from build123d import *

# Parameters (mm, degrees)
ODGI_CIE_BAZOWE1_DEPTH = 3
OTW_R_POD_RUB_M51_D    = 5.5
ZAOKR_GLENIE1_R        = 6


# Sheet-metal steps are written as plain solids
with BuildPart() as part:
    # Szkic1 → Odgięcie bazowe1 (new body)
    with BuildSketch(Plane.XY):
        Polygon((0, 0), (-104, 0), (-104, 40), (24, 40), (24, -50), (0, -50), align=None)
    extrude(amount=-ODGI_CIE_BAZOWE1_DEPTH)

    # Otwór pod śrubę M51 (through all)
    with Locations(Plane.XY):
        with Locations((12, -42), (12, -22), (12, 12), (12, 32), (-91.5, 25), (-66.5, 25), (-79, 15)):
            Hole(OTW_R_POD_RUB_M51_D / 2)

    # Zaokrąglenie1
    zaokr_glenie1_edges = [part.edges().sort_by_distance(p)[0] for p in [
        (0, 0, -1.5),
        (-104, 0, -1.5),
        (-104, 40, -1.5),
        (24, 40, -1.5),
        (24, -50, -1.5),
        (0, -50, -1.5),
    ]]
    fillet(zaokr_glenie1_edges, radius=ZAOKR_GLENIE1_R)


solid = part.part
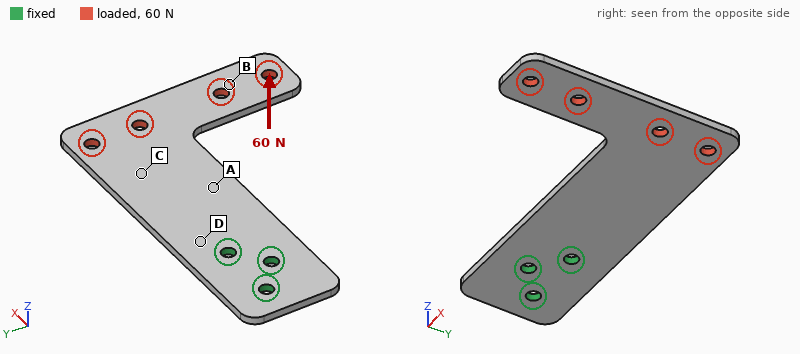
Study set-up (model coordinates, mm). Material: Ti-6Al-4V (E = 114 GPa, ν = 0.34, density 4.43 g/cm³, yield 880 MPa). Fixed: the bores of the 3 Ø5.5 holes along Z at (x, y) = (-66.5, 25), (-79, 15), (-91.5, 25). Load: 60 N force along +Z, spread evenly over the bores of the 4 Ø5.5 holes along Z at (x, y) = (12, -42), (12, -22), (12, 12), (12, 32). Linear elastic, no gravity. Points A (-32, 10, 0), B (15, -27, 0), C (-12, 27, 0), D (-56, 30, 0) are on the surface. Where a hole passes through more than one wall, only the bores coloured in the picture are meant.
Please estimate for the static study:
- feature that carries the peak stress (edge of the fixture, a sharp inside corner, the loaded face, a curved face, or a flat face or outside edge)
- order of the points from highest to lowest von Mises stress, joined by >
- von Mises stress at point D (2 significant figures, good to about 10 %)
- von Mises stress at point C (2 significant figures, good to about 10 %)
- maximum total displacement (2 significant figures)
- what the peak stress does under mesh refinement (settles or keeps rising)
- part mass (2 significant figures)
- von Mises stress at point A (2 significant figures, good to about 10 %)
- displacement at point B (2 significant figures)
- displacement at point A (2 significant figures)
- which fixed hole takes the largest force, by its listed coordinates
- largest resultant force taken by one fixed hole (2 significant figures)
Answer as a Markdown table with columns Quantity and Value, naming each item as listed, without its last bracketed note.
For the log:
| Quantity | Value |
|---|---|
| feature that carries the peak stress | edge of the fixture |
| order of the points from highest to lowest von Mises stress, joined by > | D > A > C > B |
| von Mises stress at point D | 74 MPa |
| von Mises stress at point C | 28 MPa |
| maximum total displacement | 1.9 mm |
| what the peak stress does under mesh refinement | keeps rising |
| part mass | 81 g |
| von Mises stress at point A | 48 MPa |
| displacement at point B | 1.5 mm |
| displacement at point A | 0.28 mm |
| which fixed hole takes the largest force, by its listed coordinates | (-66.5, 25) |
| largest resultant force taken by one fixed hole | 150 N |
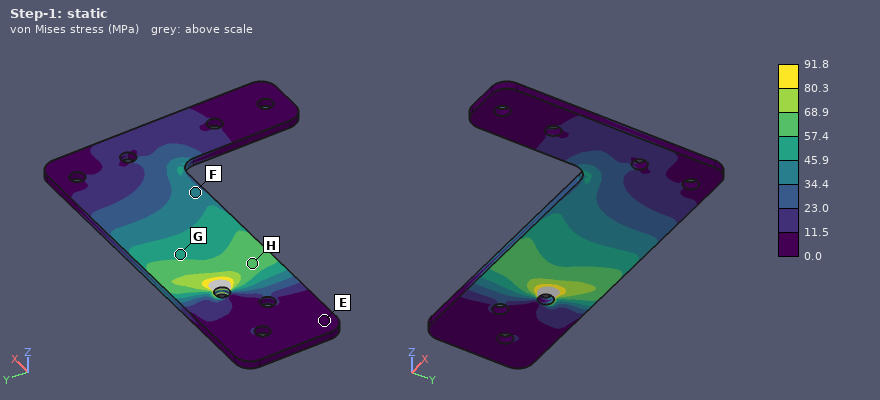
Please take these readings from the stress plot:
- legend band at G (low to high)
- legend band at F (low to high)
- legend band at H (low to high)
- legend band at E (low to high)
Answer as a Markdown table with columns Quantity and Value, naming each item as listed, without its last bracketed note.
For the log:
| Quantity | Value |
|---|---|
| legend band at G | 45.9 to 57.4 MPa |
| legend band at F | 34.4 to 45.9 MPa |
| legend band at H | 57.4 to 68.9 MPa |
| legend band at E | 0.0 to 11.5 MPa |
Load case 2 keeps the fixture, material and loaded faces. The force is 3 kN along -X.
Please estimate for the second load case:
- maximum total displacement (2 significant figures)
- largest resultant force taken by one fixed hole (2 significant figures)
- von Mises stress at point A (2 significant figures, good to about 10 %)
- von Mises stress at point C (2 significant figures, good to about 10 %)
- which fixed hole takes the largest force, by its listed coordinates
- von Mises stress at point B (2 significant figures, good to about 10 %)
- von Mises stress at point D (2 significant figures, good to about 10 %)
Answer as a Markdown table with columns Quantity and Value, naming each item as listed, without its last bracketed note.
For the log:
| Quantity | Value |
|---|---|
| maximum total displacement | 0.51 mm |
| largest resultant force taken by one fixed hole | 3.7 kN |
| von Mises stress at point A | 74 MPa |
| von Mises stress at point C | 18 MPa |
| which fixed hole takes the largest force, by its listed coordinates | (-79, 15) |
| von Mises stress at point B | 36 MPa |
| von Mises stress at point D | 22 MPa |
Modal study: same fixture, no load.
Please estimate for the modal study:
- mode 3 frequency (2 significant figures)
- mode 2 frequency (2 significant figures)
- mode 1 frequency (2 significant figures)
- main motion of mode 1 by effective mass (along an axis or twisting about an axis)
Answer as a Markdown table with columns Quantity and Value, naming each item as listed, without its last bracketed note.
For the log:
| Quantity | Value |
|---|---|
| mode 3 frequency | 1700 Hz |
| mode 2 frequency | 490 Hz |
| mode 1 frequency | 200 Hz |
| main motion of mode 1 by effective mass | along Z |
